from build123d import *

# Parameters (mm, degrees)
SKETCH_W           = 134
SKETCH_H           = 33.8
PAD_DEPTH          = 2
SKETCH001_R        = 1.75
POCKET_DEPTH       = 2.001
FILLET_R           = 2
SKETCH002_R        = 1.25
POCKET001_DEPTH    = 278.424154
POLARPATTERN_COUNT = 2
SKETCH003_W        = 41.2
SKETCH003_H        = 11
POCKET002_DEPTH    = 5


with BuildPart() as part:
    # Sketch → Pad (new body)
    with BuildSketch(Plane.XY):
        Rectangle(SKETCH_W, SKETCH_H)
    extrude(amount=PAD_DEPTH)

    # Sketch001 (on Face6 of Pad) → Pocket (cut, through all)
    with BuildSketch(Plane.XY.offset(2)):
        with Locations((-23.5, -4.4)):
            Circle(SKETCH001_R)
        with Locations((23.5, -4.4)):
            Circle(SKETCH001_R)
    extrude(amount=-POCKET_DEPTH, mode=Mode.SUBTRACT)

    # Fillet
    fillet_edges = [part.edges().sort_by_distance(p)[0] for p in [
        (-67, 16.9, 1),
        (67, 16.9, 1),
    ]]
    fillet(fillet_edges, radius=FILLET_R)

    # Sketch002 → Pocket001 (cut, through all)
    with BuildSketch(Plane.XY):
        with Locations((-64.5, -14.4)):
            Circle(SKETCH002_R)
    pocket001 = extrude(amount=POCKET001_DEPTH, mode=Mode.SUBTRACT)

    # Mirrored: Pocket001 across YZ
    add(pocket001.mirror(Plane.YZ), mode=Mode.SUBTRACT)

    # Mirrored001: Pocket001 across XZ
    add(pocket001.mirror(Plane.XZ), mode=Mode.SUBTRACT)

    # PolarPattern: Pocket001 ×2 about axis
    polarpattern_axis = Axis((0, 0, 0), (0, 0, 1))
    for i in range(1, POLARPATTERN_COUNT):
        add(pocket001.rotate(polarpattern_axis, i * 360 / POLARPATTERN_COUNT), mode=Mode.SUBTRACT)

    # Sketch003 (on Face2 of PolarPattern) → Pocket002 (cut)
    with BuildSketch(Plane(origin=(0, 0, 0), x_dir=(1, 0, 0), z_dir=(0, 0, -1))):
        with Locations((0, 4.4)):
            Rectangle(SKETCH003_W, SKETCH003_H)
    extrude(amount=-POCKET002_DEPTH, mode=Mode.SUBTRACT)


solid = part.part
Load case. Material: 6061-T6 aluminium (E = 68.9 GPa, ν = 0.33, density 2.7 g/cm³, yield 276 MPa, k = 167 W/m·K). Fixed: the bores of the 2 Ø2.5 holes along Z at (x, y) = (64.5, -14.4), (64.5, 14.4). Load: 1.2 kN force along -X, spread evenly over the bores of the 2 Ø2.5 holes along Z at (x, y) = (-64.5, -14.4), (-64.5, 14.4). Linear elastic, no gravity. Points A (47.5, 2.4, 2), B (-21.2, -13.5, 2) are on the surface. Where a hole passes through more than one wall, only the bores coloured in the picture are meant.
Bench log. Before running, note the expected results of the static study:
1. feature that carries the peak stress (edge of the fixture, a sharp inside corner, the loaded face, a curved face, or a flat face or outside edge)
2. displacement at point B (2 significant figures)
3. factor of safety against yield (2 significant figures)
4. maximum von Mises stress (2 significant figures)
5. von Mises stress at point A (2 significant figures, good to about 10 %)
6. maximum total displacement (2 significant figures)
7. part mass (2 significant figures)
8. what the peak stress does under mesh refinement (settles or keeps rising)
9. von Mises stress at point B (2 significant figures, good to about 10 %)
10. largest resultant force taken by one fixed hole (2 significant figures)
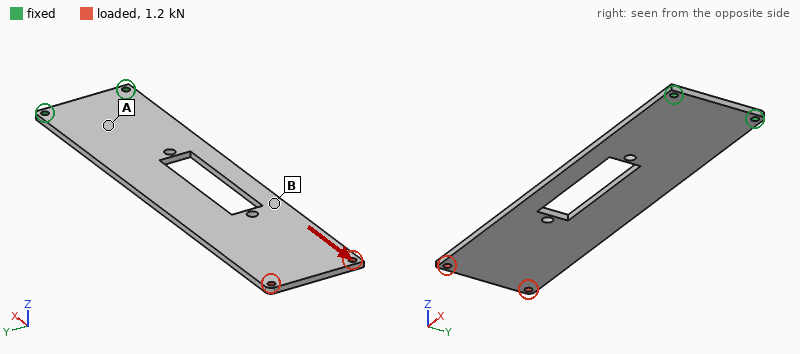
the loaded face
38 µm
1.8
150 MPa
12 MPa
66 µm
22 g
settles
31 MPa
630 N
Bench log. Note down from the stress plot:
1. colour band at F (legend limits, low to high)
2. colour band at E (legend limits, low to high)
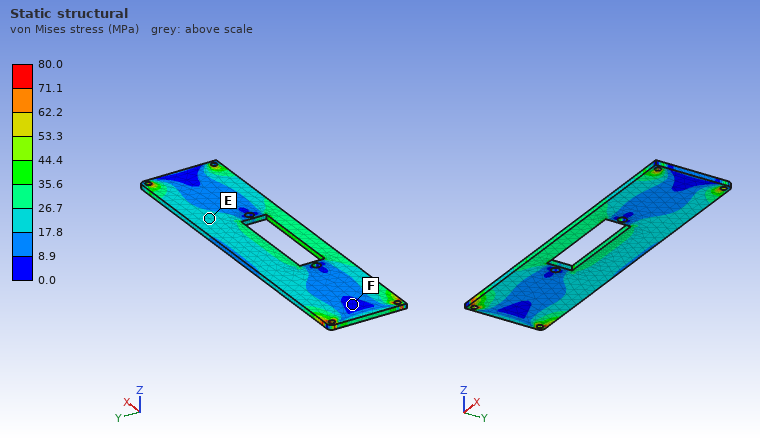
0.0 to 8.9 MPa
17.8 to 26.7 MPa
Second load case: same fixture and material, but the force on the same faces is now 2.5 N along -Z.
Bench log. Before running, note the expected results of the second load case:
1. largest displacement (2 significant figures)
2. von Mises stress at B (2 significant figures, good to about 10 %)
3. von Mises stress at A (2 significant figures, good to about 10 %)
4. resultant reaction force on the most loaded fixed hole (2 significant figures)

1.4 mm
6.5 MPa
12 MPa
1.3 N
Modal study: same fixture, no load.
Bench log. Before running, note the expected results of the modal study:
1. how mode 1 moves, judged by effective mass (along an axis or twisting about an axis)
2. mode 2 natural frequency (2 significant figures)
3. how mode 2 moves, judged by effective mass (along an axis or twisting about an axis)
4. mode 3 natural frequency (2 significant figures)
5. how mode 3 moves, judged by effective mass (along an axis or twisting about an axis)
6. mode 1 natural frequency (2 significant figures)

along Z
560 Hz
along Z
670 Hz
twisting about X
89 Hz
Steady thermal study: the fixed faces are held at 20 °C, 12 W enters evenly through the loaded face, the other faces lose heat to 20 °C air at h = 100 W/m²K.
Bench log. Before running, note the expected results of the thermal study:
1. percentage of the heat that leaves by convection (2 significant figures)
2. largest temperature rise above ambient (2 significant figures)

95 %
51 K
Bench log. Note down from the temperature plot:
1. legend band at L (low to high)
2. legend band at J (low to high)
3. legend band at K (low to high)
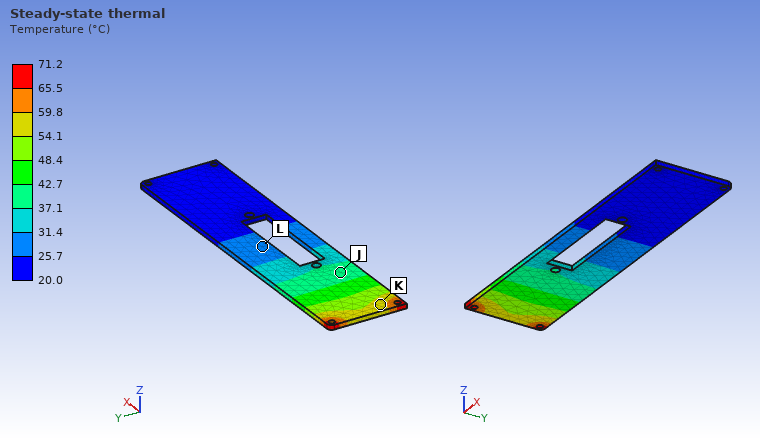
25.7 to 31.4 °C
37.1 to 42.7 °C
54.1 to 59.8 °C
